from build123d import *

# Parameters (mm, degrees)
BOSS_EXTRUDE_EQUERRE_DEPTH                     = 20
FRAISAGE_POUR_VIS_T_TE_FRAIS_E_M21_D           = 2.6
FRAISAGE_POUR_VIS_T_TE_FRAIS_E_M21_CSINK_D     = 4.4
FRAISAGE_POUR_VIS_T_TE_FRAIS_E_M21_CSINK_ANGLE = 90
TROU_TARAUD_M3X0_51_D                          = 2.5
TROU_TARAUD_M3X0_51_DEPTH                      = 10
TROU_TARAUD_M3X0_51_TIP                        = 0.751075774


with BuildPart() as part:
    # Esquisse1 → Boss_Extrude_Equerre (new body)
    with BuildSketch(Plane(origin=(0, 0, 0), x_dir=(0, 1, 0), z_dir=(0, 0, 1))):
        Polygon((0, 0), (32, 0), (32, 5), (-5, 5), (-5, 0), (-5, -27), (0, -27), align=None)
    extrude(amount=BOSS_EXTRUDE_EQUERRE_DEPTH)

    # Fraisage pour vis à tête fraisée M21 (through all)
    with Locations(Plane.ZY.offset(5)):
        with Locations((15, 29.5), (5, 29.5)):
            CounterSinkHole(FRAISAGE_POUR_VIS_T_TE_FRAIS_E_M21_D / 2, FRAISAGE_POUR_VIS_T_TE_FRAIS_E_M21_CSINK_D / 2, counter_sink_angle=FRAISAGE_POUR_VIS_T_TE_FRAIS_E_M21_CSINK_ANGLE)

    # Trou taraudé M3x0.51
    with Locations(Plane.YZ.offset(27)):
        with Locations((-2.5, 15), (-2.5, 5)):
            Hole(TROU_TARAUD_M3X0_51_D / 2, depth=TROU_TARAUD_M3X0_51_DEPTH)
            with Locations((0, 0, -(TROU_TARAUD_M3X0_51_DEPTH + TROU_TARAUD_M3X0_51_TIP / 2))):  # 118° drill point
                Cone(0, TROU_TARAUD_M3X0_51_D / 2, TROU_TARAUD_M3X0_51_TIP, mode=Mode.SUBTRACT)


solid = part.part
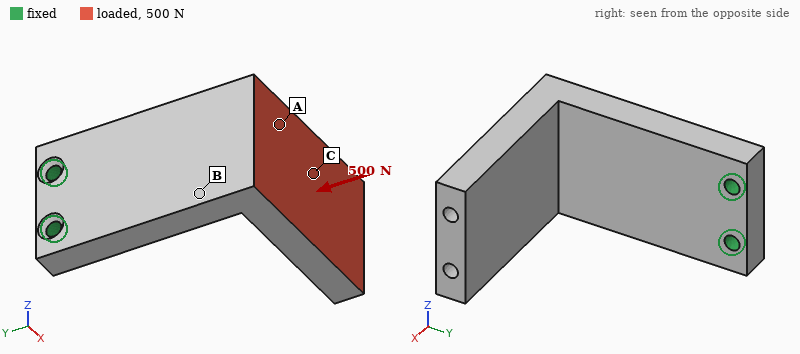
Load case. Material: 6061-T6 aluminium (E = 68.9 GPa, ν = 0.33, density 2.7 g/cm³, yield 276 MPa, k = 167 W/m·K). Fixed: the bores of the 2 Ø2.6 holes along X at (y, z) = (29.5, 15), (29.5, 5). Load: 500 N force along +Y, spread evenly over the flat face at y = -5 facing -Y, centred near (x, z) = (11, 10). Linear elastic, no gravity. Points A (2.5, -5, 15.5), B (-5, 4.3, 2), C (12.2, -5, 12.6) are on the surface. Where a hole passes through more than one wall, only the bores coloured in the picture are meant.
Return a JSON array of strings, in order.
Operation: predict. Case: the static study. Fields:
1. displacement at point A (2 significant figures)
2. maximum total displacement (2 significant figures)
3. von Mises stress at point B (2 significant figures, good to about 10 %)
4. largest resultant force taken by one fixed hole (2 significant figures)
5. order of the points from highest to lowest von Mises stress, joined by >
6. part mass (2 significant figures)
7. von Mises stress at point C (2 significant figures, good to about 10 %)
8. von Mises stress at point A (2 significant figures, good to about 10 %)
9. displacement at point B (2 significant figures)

["0.31 mm", "0.61 mm", "78 MPa", "250 N", "B > A > C", "17 g", "20 MPa", "53 MPa", "0.16 mm"]
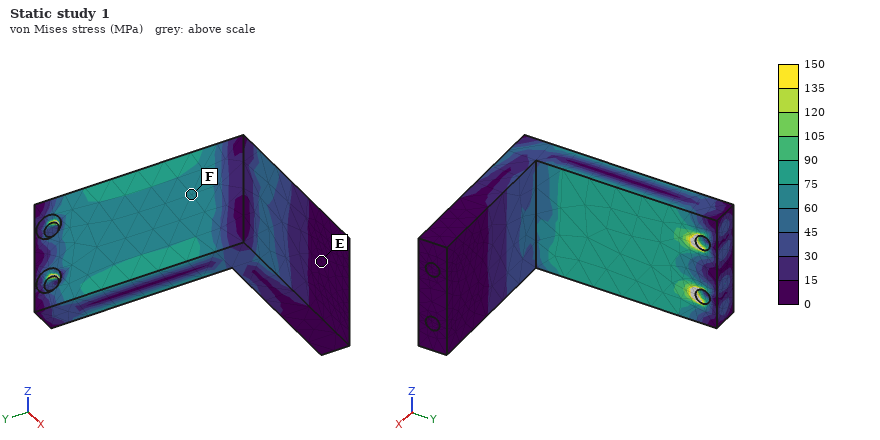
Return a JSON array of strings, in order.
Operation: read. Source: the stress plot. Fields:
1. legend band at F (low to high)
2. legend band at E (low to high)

["60 to 75 MPa", "0 to 15 MPa"]
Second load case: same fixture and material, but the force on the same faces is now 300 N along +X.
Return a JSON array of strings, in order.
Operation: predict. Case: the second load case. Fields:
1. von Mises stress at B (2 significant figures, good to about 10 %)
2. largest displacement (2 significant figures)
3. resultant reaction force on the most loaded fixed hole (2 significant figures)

["34 MPa", "0.51 mm", "150 N"]
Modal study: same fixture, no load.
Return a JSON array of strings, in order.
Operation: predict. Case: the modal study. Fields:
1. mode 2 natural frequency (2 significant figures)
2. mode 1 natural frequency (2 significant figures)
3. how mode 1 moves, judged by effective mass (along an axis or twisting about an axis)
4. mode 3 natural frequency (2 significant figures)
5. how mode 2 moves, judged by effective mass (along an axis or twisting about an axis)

["2500 Hz", "1400 Hz", "along X", "4200 Hz", "along Z"]
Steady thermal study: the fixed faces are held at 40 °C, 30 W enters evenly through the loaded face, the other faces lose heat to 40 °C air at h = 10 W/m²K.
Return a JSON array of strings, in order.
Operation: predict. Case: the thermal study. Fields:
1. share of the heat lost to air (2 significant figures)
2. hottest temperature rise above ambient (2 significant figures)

["4.1 %", "77 K"]
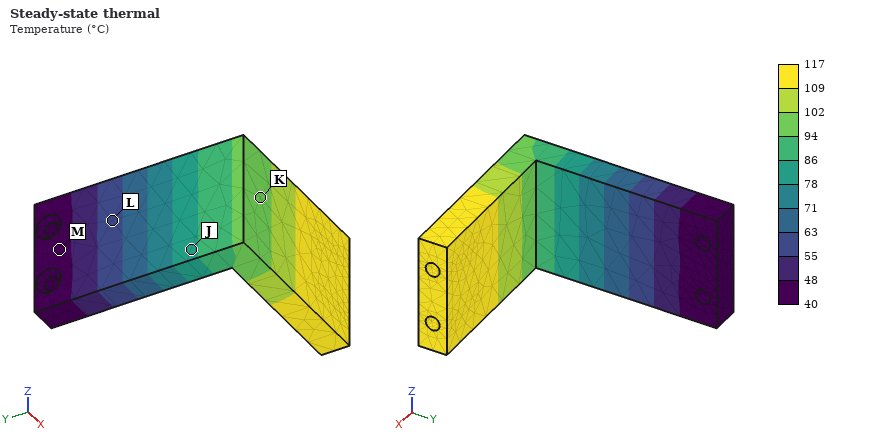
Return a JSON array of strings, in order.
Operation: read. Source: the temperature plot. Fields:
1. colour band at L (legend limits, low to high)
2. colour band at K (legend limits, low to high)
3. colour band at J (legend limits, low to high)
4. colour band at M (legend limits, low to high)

["55 to 63 °C", "94 to 102 °C", "78 to 86 °C", "40 to 48 °C"]
